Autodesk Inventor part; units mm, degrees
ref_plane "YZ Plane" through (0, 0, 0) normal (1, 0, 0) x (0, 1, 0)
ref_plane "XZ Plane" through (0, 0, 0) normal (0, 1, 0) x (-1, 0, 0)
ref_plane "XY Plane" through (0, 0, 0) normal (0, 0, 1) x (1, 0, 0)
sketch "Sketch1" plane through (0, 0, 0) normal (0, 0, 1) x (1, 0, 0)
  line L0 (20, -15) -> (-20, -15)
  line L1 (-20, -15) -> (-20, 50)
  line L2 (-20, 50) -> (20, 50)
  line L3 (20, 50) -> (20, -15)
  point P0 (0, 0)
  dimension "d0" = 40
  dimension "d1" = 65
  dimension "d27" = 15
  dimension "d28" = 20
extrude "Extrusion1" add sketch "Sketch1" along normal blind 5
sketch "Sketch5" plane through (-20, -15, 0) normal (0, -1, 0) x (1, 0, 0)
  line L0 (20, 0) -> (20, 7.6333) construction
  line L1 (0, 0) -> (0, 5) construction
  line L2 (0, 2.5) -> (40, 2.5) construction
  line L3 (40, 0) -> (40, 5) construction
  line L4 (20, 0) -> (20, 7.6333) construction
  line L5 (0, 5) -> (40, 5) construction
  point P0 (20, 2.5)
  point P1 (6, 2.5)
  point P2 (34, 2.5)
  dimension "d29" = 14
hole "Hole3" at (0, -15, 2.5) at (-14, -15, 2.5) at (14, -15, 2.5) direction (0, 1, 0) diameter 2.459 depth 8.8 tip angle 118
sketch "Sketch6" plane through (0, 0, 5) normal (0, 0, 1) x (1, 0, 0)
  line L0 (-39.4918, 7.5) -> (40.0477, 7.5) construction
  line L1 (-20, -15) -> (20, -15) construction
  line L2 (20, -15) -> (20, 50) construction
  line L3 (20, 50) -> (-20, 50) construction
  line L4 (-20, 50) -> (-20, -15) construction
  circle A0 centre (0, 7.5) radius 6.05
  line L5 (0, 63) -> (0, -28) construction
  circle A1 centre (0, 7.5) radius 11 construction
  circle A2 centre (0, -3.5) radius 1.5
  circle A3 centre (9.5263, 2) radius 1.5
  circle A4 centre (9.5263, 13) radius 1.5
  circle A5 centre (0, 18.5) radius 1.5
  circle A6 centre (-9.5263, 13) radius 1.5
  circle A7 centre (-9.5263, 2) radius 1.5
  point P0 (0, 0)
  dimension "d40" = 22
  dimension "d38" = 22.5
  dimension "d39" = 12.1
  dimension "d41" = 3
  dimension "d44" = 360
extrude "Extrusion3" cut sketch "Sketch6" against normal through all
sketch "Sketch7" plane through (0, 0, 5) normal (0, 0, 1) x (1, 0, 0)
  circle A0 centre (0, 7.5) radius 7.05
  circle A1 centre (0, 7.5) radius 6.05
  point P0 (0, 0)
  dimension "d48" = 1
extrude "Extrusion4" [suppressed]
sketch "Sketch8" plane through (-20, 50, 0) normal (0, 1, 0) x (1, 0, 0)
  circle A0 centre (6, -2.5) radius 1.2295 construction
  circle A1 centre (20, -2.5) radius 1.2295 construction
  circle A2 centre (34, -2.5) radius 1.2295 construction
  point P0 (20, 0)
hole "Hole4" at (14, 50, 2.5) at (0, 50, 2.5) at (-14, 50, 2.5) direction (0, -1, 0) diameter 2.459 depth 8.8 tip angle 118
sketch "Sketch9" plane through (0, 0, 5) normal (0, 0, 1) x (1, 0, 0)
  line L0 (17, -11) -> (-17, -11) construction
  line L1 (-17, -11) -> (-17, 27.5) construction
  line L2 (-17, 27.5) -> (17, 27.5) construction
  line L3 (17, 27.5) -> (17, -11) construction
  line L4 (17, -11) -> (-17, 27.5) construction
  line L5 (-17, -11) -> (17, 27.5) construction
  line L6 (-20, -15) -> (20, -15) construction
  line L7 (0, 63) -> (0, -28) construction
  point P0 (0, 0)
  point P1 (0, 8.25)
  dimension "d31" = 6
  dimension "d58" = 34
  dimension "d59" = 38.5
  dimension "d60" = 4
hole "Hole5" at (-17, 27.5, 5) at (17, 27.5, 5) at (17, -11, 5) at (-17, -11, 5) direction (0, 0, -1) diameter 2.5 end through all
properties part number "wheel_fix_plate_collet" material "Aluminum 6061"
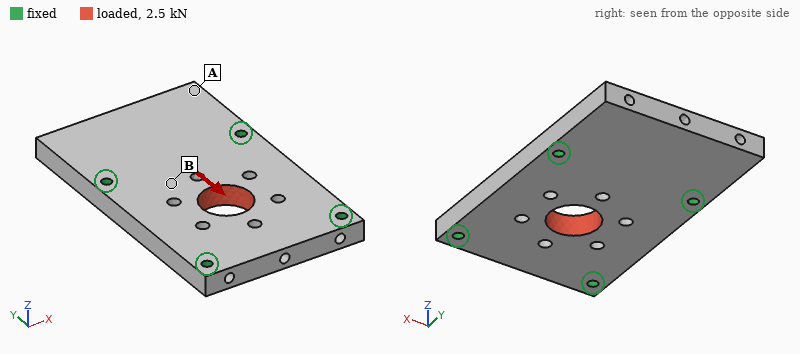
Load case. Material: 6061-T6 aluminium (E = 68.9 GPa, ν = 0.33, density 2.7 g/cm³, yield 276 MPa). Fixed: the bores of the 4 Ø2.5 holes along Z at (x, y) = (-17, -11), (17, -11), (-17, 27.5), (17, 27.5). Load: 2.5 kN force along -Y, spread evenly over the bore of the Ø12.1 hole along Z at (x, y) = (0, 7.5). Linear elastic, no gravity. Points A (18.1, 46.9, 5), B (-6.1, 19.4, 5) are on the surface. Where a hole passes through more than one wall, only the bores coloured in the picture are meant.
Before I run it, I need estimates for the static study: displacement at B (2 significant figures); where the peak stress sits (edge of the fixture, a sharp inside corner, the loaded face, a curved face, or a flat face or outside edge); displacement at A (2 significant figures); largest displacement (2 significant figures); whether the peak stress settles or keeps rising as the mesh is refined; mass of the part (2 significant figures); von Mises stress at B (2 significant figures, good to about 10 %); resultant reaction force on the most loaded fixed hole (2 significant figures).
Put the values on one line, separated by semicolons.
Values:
2.8 µm; edge of the fixture; 0.99 µm; 6.0 µm; keeps rising; 32 g; 11 MPa; 730 N
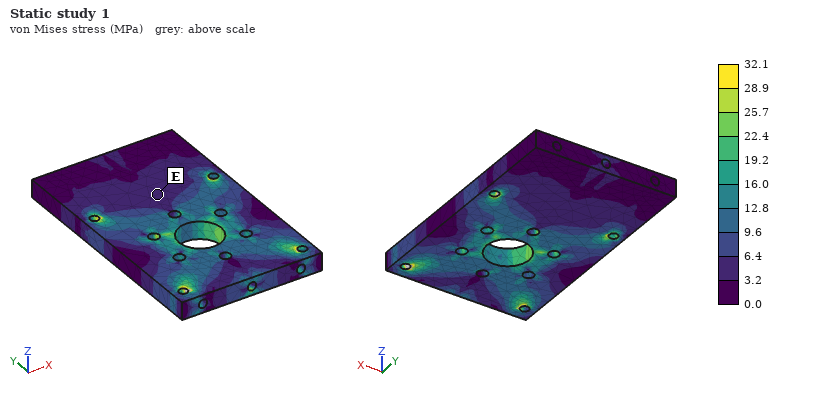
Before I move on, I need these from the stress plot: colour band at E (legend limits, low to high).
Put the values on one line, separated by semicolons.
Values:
3.2 to 6.4 MPa
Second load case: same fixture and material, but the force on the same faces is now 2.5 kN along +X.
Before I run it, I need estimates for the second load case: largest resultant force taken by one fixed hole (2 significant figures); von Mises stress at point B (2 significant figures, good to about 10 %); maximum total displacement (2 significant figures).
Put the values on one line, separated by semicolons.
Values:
740 N; 14 MPa; 7.2 µm
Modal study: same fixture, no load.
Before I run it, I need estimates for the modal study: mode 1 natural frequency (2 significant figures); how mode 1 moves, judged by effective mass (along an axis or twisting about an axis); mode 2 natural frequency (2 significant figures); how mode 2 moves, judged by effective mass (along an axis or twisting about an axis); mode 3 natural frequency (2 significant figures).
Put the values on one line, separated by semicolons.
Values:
6300 Hz; along Z; 11 kHz; along Z; 12 kHz
